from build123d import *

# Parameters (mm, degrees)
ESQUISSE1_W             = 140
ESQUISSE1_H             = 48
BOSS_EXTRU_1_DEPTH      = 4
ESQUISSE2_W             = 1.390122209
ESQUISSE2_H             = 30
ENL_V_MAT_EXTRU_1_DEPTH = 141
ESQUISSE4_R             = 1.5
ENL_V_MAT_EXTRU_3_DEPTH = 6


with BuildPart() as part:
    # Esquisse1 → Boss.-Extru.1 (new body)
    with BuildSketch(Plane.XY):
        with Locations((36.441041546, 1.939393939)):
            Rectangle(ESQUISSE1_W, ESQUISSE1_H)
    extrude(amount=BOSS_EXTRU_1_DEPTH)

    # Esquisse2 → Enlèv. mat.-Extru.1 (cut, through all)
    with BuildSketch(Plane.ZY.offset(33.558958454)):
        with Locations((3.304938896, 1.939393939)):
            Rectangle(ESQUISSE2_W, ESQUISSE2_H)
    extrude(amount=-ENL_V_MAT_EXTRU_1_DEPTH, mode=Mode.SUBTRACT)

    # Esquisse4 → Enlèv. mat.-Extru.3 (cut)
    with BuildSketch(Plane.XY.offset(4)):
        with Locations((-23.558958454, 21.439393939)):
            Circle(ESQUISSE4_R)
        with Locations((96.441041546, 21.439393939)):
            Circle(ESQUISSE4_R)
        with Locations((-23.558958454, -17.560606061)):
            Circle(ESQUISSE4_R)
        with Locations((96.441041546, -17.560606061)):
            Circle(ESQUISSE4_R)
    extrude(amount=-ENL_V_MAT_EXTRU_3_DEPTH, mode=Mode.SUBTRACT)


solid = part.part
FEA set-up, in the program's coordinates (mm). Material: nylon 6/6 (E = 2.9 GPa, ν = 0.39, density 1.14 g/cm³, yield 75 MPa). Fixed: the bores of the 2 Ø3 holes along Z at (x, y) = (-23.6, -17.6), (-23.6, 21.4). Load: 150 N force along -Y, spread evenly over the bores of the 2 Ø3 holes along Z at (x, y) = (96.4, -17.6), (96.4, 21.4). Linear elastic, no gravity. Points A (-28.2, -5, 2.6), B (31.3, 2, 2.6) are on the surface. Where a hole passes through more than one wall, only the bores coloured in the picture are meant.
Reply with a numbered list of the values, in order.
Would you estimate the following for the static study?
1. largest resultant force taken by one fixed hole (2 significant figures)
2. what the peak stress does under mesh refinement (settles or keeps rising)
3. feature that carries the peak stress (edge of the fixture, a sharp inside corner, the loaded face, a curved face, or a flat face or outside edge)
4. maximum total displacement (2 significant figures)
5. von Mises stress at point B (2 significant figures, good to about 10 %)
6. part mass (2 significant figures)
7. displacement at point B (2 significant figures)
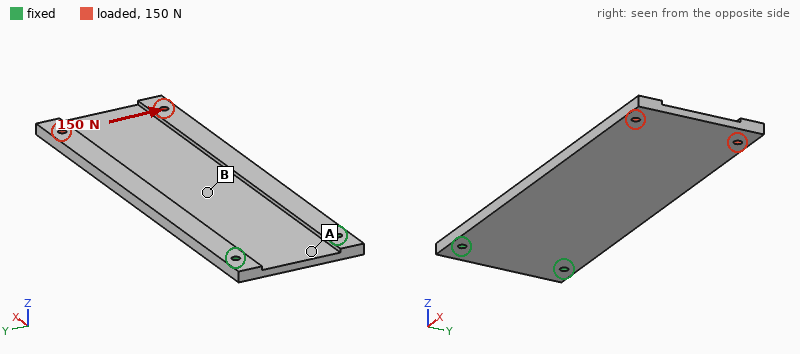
1. 460 N
2. keeps rising
3. edge of the fixture
4. 1.5 mm
5. 4.4 MPa
6. 24 g
7. 0.33 mm
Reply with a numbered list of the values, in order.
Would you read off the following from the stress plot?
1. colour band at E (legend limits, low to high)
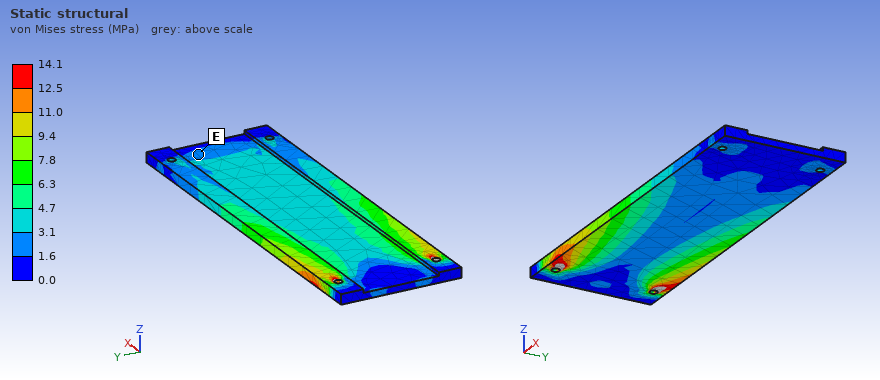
1. 1.6 to 3.1 MPa
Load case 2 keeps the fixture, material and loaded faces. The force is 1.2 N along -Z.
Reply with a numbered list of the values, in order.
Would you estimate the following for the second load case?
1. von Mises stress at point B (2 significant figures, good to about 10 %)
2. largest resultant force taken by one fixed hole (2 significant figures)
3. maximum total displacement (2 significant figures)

1. 0.46 MPa
2. 1.9 N
3. 1.7 mm
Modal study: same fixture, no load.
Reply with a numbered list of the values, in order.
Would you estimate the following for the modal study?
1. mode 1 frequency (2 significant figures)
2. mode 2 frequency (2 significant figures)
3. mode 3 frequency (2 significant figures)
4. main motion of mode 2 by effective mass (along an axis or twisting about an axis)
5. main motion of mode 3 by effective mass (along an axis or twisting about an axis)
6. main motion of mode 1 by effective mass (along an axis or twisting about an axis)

1. 54 Hz
2. 250 Hz
3. 340 Hz
4. twisting about X
5. along Z
6. along Z
